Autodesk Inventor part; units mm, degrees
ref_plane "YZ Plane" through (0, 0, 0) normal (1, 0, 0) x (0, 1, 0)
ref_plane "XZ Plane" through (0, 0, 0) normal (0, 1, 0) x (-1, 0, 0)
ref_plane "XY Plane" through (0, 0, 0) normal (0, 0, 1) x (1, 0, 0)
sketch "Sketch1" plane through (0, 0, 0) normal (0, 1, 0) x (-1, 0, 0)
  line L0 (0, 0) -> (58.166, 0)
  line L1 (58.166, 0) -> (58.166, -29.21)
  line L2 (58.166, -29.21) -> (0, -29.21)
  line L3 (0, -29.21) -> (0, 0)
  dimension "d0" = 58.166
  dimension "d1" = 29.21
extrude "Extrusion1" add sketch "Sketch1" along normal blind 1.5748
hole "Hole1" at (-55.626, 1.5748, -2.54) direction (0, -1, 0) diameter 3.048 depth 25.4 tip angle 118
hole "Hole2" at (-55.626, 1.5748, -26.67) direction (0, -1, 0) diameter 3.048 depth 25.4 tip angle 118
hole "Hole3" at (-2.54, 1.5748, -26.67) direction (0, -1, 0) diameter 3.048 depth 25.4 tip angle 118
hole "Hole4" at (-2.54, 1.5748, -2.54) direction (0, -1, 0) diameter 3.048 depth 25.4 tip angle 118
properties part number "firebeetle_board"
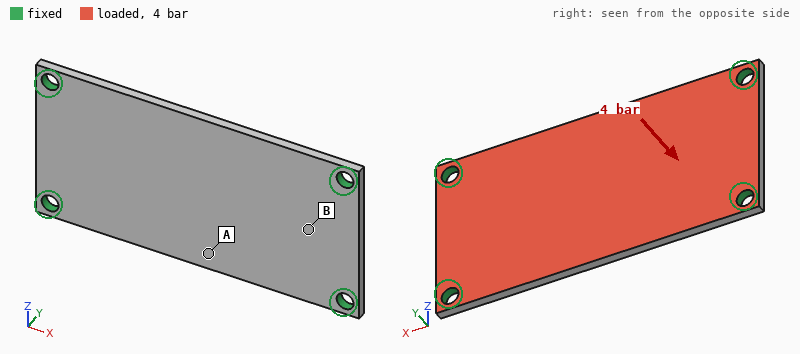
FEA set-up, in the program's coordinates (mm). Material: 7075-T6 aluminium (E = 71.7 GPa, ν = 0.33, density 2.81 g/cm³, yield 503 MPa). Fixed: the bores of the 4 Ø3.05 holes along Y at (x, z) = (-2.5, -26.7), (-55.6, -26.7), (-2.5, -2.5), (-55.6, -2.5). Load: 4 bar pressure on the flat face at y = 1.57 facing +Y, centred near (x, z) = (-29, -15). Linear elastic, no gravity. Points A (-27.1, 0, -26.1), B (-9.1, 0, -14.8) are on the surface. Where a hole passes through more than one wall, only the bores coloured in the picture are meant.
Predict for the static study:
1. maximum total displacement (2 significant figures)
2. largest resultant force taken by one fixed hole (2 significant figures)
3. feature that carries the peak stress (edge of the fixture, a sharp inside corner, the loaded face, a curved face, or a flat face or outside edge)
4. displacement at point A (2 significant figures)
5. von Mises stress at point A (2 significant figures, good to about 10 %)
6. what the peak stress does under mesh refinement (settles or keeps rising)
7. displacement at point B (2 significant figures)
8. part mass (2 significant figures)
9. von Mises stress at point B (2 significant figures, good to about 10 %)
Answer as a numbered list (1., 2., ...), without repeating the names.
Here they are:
1. 0.40 mm
2. 170 N
3. edge of the fixture
4. 0.38 mm
5. 120 MPa
6. keeps rising
7. 0.11 mm
8. 7.4 g
9. 57 MPa
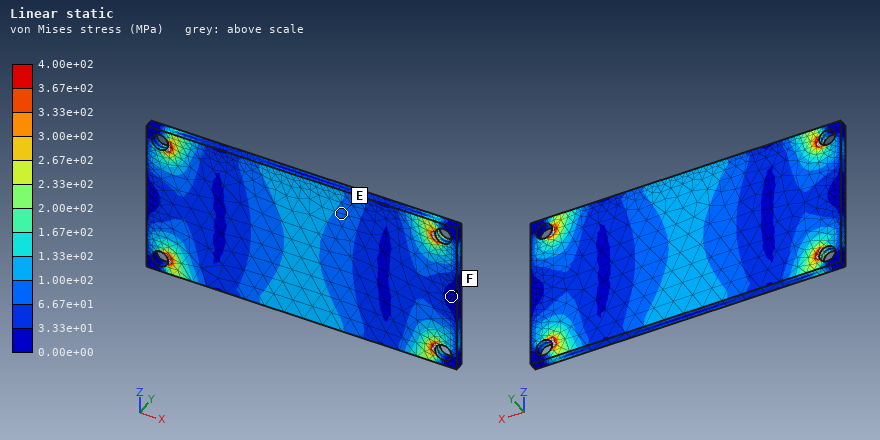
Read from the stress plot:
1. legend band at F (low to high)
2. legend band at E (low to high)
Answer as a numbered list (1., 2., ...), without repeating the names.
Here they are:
1. 0.00e+00 to 3.33e+01 MPa
2. 6.67e+01 to 1.00e+02 MPa
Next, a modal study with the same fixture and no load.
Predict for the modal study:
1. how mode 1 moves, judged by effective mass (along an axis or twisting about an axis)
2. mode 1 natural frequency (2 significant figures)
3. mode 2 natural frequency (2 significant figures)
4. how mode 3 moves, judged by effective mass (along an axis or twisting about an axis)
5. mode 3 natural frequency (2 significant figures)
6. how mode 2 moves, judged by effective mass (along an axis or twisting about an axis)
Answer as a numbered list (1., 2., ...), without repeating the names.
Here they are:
1. along Y
2. 2800 Hz
3. 4700 Hz
4. twisting about Z
5. 7600 Hz
6. twisting about X
